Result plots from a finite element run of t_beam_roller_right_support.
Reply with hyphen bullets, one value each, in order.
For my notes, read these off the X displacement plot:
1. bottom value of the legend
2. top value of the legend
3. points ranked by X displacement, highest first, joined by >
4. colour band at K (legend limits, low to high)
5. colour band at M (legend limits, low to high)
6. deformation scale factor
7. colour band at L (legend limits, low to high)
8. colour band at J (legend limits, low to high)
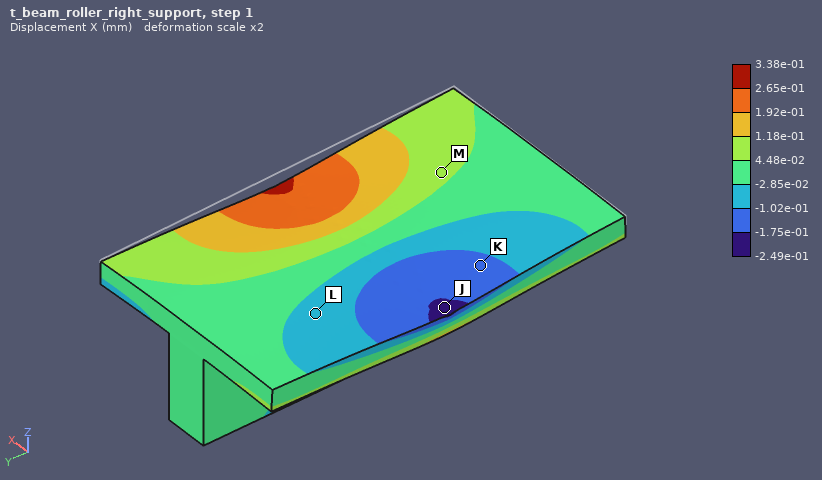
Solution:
- -2.49e-01 mm
- 3.38e-01 mm
- M > L > K > J
- -1.75e-01 to -1.02e-01 mm
- 4.48e-02 to 1.18e-01 mm
- 2
- -1.02e-01 to -2.85e-02 mm
- -2.49e-01 to -1.75e-01 mm
